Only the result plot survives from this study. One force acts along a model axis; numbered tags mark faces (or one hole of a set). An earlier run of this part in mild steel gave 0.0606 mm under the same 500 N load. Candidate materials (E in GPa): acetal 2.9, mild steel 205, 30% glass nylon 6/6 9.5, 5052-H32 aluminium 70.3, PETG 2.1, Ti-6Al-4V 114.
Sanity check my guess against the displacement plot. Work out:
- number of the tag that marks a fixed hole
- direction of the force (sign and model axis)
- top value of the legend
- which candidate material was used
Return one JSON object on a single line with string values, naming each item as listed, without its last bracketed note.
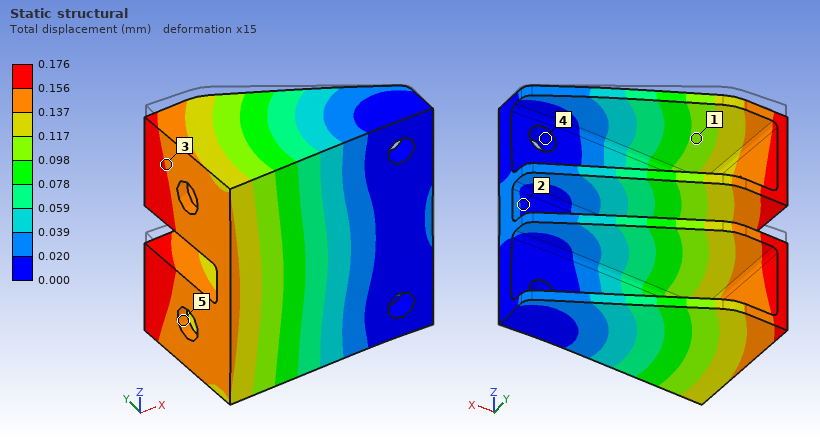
{"number of the tag that marks a fixed hole": "4", "direction of the force": "-Y", "top value of the legend": "0.176 mm", "which candidate material was used": "5052-H32 aluminium"}
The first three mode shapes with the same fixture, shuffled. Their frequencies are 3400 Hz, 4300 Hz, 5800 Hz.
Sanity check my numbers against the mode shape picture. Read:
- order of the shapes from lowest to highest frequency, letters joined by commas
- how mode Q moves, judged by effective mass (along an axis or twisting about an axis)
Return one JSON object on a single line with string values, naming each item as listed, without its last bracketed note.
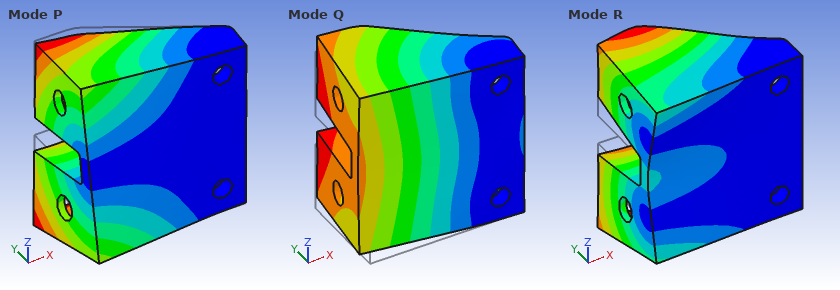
{"order of the shapes from lowest to highest frequency, letters joined by commas": "Q, P, R", "how mode Q moves, judged by effective mass": "along Y"}
